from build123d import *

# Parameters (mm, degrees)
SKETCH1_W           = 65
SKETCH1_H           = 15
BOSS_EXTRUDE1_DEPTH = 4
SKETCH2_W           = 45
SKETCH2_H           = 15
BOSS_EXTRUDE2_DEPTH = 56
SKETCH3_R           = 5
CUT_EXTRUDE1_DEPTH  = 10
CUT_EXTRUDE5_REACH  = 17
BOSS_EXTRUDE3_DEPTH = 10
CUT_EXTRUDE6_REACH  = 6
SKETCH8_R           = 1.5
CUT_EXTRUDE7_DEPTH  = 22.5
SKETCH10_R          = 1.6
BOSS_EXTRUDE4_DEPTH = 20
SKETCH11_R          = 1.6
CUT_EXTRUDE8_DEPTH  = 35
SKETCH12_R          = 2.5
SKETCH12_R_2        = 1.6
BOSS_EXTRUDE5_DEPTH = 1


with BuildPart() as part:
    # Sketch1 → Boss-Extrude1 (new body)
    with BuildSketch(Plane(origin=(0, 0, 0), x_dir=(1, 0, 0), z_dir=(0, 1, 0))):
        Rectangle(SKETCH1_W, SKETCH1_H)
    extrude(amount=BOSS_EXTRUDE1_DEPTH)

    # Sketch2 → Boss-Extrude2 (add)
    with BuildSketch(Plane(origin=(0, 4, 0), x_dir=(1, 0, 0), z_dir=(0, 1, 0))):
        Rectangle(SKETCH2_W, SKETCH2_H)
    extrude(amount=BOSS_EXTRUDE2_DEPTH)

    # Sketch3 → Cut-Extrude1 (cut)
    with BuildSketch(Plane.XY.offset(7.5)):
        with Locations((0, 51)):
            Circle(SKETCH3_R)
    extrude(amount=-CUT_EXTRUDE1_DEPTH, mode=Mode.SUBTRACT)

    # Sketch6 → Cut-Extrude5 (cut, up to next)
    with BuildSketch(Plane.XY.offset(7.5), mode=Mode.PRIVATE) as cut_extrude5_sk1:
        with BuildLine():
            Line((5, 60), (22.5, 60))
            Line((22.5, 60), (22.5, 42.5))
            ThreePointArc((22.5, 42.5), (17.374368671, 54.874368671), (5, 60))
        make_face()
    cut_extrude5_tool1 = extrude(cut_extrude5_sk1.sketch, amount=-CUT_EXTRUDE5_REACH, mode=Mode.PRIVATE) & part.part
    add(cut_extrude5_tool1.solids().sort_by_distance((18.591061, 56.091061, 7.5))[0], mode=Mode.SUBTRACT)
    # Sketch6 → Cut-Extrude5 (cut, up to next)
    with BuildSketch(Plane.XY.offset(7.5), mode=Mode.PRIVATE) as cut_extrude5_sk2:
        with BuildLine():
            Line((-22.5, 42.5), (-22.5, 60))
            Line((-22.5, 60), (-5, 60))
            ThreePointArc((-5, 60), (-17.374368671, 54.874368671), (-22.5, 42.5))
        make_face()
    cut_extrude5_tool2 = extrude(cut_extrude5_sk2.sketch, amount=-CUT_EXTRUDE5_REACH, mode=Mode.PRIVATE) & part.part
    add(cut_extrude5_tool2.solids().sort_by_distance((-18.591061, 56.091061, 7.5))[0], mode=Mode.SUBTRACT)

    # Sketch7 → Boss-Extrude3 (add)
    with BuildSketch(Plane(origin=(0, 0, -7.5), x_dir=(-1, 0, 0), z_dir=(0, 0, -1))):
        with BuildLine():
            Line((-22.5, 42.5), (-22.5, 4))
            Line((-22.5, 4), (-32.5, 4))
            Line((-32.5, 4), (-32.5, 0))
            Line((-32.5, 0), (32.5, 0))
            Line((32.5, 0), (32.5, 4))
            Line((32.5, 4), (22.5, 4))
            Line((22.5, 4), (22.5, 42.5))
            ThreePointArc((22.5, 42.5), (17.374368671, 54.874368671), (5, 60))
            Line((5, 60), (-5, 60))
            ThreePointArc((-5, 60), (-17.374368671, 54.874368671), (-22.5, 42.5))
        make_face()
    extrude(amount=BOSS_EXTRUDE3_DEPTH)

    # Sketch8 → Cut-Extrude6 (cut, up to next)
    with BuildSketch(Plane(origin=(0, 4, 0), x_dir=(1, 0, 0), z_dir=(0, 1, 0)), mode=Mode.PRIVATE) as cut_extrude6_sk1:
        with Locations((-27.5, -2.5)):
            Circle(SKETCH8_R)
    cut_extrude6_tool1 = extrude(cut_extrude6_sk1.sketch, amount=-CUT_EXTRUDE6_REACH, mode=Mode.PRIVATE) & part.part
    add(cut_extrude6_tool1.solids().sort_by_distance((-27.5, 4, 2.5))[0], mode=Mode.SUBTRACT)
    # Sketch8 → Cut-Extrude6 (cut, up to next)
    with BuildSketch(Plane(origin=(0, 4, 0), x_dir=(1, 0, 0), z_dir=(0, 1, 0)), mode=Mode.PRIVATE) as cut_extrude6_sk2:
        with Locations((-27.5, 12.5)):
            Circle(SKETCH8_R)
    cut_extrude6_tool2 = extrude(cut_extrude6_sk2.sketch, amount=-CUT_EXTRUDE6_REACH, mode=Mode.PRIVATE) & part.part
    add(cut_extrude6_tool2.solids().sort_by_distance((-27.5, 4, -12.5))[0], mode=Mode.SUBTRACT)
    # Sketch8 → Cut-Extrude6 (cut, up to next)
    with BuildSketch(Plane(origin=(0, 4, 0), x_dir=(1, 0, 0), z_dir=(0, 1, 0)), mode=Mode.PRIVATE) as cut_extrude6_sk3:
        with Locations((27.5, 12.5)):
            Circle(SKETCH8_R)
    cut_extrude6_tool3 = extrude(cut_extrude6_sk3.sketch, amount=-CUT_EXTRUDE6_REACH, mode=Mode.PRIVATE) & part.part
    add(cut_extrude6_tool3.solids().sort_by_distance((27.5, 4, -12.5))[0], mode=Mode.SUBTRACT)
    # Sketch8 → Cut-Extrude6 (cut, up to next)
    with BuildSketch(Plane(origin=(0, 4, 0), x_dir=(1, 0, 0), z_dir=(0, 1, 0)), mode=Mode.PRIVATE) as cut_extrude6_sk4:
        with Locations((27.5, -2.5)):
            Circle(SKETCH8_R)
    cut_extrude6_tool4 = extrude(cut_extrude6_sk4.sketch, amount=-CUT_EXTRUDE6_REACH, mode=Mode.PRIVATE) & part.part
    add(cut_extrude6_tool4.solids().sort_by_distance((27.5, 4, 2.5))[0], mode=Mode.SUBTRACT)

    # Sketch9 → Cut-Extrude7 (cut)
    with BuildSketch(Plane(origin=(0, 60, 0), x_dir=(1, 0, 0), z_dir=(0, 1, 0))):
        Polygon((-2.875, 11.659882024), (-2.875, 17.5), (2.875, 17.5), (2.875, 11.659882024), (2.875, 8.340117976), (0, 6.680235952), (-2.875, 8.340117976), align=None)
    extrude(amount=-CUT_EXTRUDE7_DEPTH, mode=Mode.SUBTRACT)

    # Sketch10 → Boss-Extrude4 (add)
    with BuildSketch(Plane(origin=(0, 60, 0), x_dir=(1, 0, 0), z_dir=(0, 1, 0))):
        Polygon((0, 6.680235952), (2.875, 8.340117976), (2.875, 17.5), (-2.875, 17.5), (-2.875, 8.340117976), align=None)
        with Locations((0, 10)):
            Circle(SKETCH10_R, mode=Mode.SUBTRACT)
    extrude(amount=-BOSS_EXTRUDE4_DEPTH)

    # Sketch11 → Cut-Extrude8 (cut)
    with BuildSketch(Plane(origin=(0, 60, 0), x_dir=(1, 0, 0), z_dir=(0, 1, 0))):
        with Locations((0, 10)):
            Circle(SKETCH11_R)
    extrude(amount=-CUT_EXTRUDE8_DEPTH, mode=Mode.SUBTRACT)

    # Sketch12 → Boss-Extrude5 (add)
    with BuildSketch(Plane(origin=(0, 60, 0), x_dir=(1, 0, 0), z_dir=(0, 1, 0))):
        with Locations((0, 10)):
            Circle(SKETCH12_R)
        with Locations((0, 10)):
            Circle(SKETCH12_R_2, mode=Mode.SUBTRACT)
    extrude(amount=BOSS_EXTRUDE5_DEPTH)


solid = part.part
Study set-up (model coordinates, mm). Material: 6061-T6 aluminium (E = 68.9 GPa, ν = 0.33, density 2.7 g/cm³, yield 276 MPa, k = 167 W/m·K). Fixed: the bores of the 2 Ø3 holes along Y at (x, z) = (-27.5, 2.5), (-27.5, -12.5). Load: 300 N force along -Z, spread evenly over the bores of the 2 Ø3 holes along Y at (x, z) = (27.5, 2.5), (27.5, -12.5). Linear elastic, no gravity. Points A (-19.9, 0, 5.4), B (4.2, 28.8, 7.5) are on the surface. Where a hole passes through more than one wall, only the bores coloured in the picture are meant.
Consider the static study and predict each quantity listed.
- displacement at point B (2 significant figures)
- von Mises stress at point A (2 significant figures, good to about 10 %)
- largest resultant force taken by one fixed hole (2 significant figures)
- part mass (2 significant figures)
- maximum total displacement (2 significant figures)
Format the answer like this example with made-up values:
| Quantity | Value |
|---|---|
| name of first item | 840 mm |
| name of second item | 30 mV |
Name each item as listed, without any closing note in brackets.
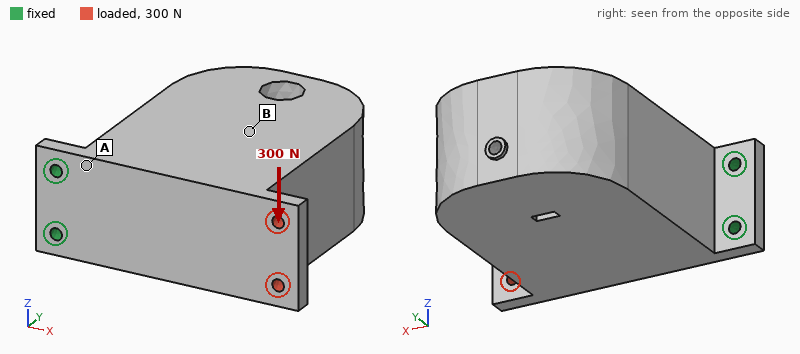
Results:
| Quantity | Value |
|---|---|
| displacement at point B | 15 µm |
| von Mises stress at point A | 25 MPa |
| largest resultant force taken by one fixed hole | 1.0 kN |
| part mass | 180 g |
| maximum total displacement | 43 µm |
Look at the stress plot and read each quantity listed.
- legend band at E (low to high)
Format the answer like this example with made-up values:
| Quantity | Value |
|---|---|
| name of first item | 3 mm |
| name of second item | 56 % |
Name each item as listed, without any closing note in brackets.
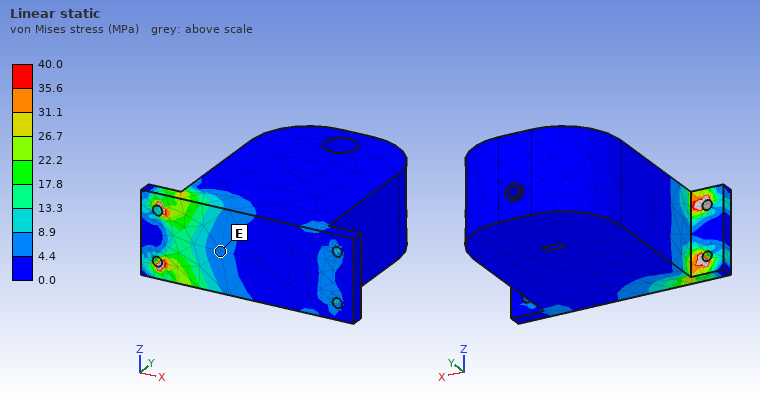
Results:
| Quantity | Value |
|---|---|
| legend band at E | 4.4 to 8.9 MPa |
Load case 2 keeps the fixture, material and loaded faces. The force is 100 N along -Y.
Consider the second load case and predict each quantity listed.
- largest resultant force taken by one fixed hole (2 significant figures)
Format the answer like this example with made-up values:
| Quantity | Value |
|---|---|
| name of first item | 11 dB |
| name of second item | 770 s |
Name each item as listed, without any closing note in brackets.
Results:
| Quantity | Value |
|---|---|
| largest resultant force taken by one fixed hole | 50 N |
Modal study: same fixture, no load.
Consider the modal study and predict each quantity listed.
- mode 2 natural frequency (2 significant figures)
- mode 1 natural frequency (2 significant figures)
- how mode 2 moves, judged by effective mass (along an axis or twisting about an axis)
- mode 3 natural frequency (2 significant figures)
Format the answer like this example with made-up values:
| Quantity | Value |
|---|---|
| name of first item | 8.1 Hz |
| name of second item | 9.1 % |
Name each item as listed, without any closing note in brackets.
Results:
| Quantity | Value |
|---|---|
| mode 2 natural frequency | 1100 Hz |
| mode 1 natural frequency | 340 Hz |
| how mode 2 moves, judged by effective mass | along Z |
| mode 3 natural frequency | 2800 Hz |
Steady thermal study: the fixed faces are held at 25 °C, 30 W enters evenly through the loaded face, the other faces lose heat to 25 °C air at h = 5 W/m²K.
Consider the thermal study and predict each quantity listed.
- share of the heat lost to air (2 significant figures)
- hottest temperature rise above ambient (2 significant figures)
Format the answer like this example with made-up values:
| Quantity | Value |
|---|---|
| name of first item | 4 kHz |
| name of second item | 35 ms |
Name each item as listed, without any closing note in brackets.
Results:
| Quantity | Value |
|---|---|
| share of the heat lost to air | 4.2 % |
| hottest temperature rise above ambient | 47 K |
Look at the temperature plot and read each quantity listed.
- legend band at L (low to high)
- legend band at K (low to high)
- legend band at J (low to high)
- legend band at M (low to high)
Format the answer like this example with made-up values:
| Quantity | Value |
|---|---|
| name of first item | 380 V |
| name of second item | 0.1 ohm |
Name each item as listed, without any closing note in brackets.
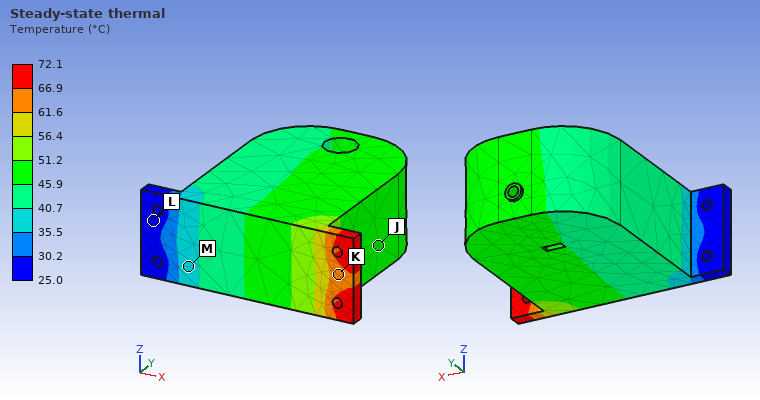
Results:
| Quantity | Value |
|---|---|
| legend band at L | 25.0 to 30.2 °C |
| legend band at K | 61.6 to 66.9 °C |
| legend band at J | 45.9 to 51.2 °C |
| legend band at M | 35.5 to 40.7 °C |
